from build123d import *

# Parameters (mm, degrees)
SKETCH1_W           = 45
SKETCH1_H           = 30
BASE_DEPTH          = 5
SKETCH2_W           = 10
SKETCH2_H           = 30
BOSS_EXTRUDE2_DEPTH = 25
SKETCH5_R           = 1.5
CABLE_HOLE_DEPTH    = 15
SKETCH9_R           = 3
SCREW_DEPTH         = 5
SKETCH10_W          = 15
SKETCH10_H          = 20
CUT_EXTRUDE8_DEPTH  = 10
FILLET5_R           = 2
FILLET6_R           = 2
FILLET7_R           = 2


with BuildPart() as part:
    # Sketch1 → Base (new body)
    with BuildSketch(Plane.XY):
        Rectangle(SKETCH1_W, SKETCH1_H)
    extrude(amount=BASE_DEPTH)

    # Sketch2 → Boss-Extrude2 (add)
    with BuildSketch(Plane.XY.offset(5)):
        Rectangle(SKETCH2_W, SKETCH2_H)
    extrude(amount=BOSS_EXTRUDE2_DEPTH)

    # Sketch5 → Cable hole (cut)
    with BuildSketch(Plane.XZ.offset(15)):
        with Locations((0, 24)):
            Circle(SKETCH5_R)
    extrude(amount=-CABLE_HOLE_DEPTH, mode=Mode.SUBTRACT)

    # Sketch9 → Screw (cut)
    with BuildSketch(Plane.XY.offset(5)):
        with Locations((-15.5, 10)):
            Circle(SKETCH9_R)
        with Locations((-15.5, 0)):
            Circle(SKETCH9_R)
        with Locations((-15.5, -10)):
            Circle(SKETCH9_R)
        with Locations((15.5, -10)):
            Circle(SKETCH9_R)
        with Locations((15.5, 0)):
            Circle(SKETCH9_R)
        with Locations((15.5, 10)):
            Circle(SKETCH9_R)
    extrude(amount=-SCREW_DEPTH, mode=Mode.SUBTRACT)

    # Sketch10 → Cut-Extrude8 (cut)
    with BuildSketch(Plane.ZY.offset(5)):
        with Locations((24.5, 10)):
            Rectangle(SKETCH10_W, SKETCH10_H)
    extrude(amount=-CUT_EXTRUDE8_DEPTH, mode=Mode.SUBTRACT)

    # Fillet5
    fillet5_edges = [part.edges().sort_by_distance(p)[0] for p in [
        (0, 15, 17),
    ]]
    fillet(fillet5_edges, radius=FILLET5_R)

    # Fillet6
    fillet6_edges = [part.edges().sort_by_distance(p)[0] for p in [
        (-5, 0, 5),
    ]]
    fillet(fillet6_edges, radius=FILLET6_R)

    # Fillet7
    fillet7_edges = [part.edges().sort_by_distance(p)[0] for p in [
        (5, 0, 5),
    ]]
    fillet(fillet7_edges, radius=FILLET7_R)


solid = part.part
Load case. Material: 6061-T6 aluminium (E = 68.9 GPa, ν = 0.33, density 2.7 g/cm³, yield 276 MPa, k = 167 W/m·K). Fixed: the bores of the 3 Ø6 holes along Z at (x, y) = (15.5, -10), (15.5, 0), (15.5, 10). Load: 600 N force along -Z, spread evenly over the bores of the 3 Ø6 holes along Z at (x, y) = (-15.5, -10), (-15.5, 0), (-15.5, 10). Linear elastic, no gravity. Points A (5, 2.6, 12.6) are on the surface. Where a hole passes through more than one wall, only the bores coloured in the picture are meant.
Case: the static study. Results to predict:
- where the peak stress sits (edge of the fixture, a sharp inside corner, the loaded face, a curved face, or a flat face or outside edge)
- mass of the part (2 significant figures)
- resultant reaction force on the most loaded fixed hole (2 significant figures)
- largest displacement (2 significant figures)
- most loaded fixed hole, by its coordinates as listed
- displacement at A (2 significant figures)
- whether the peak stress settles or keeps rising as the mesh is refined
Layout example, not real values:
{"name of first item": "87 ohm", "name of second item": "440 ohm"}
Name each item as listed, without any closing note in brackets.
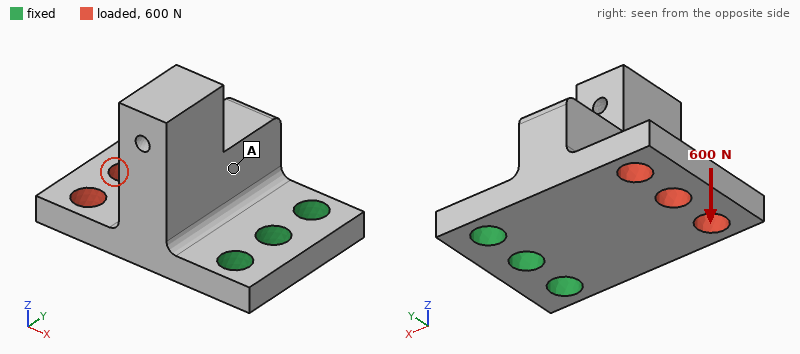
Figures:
{"where the peak stress sits": "edge of the fixture", "mass of the part": "31 g", "resultant reaction force on the most loaded fixed hole": "250 N", "largest displacement": "0.23 mm", "most loaded fixed hole, by its coordinates as listed": "(15.5, 0)", "displacement at A": "0.066 mm", "whether the peak stress settles or keeps rising as the mesh is refined": "keeps rising"}
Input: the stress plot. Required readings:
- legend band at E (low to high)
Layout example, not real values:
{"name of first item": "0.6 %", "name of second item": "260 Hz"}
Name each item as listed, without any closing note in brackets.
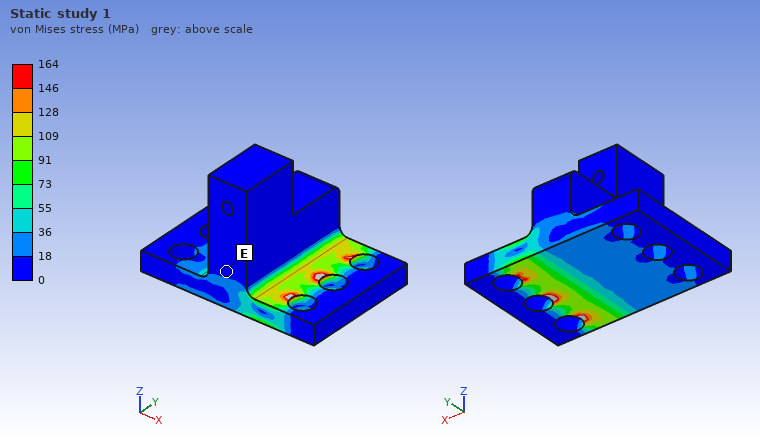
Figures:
{"legend band at E": "0 to 18 MPa"}
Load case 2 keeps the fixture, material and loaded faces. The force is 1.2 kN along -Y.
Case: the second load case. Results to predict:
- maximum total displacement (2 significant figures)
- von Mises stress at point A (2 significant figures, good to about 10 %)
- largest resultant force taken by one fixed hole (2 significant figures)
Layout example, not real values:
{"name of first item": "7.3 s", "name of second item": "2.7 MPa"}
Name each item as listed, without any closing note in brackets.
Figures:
{"maximum total displacement": "33 µm", "von Mises stress at point A": "4.7 MPa", "largest resultant force taken by one fixed hole": "1.6 kN"}
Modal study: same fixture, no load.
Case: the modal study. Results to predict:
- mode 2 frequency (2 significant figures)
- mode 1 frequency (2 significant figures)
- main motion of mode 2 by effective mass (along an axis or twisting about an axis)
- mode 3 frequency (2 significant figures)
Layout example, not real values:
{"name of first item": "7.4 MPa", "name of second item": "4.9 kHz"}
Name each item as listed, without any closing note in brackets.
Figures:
{"mode 2 frequency": "7000 Hz", "mode 1 frequency": "2700 Hz", "main motion of mode 2 by effective mass": "along Y", "mode 3 frequency": "11 kHz"}
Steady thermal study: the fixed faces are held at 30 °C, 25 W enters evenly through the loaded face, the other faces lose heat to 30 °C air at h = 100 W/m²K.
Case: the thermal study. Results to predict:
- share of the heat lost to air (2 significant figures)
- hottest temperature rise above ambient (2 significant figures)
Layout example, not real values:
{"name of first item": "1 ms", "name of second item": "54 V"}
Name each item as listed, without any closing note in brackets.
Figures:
{"share of the heat lost to air": "19 %", "hottest temperature rise above ambient": "26 K"}
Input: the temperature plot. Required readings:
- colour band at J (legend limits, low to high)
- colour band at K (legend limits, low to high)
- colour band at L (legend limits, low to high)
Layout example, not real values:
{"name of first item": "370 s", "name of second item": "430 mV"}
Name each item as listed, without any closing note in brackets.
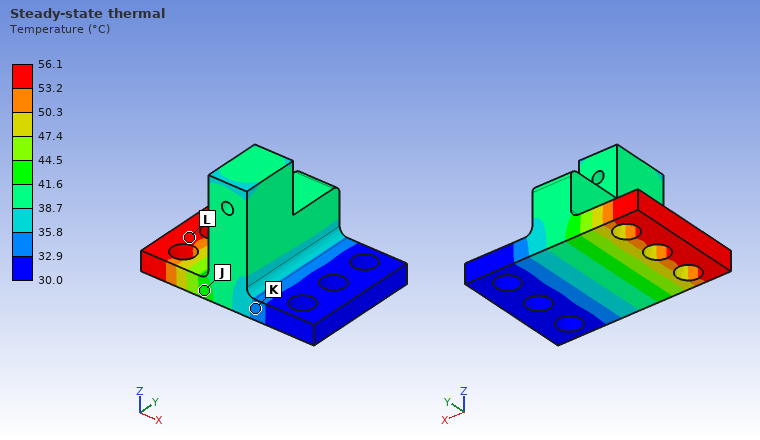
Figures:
{"colour band at J": "41.6 to 44.5 °C", "colour band at K": "32.9 to 35.8 °C", "colour band at L": "53.2 to 56.1 °C"}
